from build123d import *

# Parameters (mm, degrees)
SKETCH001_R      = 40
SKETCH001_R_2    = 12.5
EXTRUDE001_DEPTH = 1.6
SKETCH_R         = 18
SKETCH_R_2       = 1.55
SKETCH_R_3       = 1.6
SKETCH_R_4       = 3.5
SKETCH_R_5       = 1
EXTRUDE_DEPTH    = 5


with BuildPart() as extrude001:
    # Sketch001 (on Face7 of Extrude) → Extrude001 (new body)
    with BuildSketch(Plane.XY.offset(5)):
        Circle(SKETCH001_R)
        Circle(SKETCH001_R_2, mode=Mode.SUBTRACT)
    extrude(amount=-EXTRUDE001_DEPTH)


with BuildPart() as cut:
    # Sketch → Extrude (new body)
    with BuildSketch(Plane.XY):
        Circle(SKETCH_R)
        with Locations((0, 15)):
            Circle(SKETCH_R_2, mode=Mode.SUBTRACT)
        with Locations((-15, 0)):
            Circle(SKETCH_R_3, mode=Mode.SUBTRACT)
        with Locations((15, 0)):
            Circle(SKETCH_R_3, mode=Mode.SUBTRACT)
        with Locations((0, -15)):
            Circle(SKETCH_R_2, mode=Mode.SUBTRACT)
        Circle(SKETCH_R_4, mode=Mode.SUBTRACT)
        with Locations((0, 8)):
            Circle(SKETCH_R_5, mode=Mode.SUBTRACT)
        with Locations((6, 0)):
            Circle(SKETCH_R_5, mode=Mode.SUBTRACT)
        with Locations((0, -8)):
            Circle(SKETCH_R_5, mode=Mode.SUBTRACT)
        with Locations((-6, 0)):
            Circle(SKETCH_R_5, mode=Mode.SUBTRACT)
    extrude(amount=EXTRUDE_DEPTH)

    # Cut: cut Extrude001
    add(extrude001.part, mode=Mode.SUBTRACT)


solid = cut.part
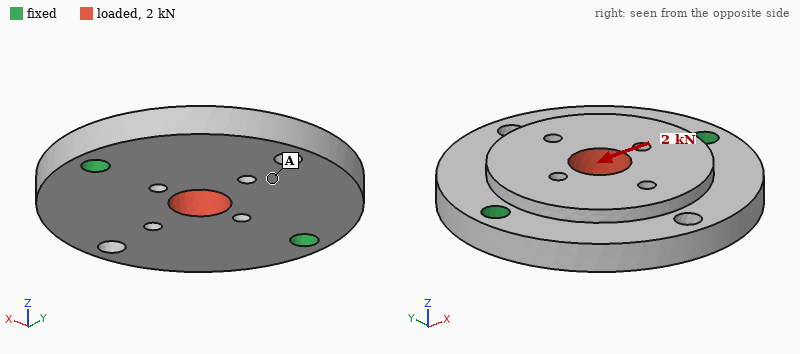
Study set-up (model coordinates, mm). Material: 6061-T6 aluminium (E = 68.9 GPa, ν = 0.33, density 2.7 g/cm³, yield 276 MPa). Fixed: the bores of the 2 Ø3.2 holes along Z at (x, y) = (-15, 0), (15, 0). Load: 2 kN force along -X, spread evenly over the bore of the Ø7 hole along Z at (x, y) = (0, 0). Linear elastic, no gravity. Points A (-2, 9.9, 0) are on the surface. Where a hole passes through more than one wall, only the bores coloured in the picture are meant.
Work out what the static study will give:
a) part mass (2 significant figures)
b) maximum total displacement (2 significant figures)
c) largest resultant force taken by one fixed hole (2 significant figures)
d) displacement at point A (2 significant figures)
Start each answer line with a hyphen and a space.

- 10 g
- 5.0 µm
- 1.0 kN
- 3.3 µm
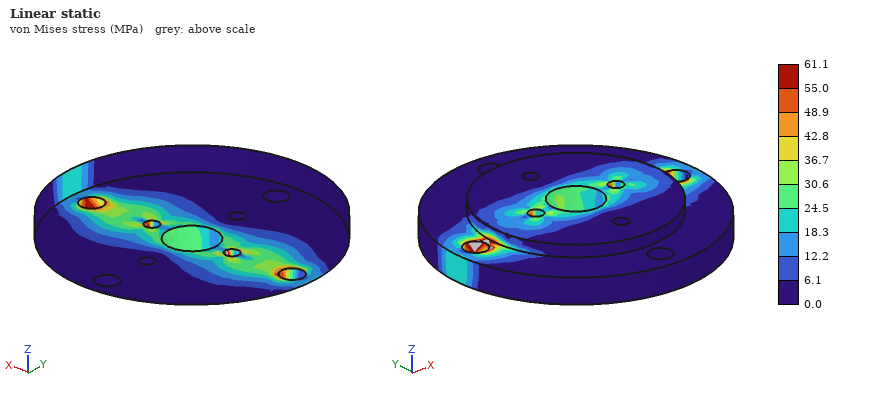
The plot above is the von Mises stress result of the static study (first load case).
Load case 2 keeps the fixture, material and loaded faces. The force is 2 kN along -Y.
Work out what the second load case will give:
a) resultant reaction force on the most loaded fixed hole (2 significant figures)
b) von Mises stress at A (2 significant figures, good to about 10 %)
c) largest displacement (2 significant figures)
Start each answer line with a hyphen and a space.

- 1.0 kN
- 22 MPa
- 15 µm
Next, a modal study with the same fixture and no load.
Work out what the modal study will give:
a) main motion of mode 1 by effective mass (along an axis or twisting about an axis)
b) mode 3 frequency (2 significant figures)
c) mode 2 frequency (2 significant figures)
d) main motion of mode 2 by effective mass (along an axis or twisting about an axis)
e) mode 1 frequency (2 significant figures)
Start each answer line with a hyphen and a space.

- twisting about X
- 24 kHz
- 12 kHz
- along Z
- 8000 Hz
